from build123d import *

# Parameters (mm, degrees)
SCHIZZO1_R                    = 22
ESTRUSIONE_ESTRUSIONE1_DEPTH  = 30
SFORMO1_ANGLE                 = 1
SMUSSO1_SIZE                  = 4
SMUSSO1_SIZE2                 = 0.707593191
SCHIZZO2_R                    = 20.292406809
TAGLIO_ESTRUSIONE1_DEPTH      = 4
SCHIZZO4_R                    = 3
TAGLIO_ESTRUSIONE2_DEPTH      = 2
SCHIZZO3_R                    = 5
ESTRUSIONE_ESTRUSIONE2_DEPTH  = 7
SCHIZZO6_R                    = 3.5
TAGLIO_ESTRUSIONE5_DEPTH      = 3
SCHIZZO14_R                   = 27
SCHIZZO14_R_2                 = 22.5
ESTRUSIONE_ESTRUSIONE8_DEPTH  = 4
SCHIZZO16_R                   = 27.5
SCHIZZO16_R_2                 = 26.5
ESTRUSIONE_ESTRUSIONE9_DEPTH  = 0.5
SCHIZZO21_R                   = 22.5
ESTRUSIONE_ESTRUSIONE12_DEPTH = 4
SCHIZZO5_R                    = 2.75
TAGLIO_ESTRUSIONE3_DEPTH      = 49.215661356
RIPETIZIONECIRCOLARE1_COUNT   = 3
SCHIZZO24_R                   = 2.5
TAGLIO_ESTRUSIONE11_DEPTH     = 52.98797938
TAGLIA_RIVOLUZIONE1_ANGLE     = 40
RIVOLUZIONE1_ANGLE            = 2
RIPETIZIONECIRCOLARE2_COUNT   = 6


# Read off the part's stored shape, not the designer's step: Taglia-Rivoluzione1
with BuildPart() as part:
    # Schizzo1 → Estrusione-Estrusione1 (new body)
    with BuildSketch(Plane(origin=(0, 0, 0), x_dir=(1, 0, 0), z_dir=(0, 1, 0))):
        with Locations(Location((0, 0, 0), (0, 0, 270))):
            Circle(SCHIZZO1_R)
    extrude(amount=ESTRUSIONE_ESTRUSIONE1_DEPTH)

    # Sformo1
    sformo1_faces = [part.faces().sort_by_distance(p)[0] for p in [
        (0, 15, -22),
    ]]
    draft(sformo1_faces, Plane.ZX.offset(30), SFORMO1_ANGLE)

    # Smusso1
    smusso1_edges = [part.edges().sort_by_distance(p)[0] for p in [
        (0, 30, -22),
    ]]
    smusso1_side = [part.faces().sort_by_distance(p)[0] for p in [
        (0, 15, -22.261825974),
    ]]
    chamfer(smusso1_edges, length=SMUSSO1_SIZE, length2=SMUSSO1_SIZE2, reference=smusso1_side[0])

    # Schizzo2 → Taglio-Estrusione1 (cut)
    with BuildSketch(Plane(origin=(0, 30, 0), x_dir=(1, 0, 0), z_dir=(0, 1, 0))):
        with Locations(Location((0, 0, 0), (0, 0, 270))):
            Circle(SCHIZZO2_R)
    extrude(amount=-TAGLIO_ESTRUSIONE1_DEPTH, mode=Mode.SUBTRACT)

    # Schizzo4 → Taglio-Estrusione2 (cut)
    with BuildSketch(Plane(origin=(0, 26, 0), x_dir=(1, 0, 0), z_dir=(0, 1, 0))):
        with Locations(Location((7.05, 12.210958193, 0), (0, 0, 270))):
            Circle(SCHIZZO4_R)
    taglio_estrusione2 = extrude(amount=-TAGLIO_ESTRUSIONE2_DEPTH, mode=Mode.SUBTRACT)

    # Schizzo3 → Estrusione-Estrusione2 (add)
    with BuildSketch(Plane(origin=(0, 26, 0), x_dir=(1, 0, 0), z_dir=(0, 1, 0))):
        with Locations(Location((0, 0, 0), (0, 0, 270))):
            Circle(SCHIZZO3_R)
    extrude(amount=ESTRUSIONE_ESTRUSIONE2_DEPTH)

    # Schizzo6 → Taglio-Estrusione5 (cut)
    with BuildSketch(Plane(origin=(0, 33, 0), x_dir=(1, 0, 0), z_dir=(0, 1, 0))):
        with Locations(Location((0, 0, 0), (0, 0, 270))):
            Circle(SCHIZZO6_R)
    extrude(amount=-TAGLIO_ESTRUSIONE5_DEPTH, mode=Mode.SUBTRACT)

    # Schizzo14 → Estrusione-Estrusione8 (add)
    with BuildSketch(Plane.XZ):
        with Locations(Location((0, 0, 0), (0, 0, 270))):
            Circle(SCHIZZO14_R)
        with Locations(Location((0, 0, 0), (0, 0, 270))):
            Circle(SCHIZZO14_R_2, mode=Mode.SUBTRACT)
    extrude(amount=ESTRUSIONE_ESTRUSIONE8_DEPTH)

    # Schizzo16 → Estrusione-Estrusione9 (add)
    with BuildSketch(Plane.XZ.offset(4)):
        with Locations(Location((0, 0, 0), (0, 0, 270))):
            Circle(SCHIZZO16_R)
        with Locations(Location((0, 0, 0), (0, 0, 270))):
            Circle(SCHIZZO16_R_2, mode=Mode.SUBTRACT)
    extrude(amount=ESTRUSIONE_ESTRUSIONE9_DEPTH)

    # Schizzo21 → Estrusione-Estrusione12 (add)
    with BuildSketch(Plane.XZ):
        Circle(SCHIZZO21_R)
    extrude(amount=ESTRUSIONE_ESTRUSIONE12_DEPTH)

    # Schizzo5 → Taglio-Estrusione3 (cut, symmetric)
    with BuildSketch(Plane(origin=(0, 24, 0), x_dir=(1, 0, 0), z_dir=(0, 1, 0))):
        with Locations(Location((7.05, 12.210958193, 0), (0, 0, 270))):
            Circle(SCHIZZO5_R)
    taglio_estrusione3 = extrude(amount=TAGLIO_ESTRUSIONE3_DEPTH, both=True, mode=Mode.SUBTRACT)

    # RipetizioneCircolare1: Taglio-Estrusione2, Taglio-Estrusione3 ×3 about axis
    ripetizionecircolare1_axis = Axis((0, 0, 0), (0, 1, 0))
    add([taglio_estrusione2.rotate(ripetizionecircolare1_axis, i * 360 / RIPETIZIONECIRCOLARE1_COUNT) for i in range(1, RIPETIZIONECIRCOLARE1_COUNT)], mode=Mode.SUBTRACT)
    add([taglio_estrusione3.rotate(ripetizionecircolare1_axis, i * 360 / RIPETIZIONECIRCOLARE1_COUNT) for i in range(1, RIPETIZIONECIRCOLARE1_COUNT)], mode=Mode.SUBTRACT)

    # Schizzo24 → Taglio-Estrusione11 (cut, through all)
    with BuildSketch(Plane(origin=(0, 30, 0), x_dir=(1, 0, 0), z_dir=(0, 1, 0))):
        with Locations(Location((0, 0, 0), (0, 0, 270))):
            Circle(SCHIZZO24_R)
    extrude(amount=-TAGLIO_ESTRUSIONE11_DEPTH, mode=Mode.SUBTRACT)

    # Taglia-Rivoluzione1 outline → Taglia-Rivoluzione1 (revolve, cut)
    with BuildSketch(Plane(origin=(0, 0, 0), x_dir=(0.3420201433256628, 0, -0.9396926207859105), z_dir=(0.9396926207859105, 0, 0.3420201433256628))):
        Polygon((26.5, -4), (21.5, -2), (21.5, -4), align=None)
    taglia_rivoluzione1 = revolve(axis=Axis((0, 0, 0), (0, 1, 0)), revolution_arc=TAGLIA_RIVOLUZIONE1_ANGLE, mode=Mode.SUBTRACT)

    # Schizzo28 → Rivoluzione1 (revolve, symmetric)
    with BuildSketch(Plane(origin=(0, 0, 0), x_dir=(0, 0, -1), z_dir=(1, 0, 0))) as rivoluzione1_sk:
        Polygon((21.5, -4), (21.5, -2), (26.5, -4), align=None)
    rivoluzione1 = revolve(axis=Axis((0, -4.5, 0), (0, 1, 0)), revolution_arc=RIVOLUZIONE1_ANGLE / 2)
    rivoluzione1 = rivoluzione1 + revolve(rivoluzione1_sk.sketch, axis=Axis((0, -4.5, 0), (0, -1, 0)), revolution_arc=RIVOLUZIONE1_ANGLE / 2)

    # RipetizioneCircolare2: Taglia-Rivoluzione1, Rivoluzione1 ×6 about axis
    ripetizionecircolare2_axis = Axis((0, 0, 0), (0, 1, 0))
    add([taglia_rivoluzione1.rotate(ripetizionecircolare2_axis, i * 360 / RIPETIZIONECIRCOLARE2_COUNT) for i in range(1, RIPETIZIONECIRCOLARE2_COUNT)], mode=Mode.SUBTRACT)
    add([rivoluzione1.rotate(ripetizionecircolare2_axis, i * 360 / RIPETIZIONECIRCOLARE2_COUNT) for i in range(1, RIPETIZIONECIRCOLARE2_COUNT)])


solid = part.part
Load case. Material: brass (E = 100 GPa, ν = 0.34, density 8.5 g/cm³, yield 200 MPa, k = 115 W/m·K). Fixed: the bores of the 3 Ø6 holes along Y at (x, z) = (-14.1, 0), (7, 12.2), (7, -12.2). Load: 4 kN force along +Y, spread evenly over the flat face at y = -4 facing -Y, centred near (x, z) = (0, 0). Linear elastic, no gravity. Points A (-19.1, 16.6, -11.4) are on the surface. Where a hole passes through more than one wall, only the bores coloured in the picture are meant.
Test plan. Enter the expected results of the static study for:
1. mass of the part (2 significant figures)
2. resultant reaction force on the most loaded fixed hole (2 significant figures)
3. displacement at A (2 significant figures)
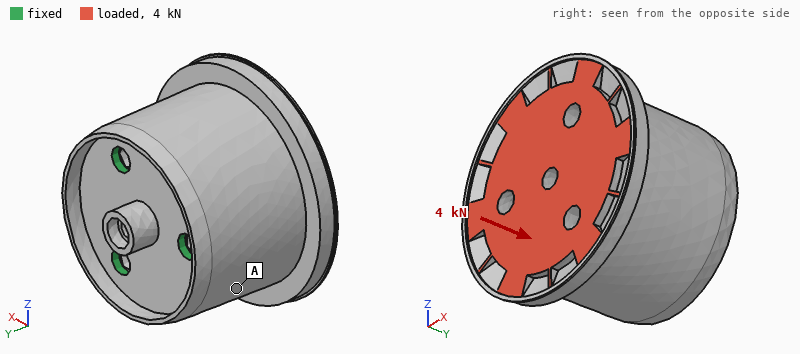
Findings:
410 g
1.3 kN
1.5 µm
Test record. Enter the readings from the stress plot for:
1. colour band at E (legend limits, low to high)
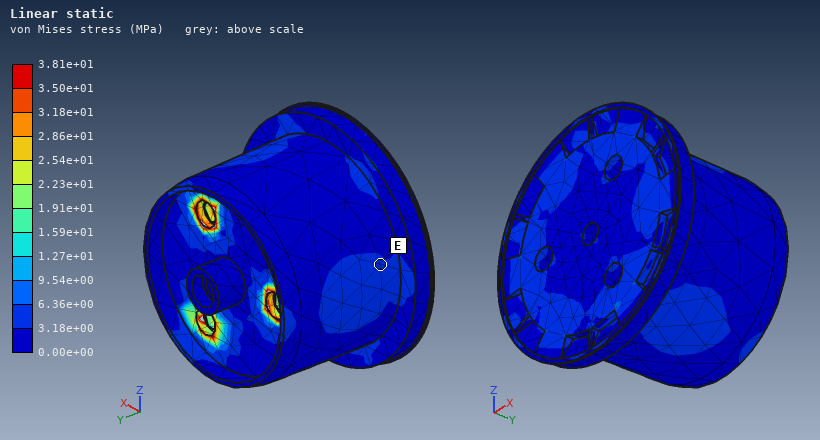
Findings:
3.18e+00 to 6.36e+00 MPa
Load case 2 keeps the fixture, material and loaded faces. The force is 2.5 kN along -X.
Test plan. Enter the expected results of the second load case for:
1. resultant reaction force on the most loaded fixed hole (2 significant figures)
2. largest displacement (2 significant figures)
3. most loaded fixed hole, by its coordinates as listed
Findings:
3.3 kN
14 µm
(-14.1, 0)
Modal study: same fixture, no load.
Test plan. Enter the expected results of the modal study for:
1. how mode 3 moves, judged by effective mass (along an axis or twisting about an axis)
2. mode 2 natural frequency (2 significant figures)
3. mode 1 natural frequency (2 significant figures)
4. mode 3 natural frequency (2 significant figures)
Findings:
twisting about Y
5900 Hz
5900 Hz
11 kHz
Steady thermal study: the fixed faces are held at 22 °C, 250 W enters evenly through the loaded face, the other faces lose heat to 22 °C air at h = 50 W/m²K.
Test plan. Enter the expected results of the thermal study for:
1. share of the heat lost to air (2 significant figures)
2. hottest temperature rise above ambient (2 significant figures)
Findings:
8.8 %
64 K
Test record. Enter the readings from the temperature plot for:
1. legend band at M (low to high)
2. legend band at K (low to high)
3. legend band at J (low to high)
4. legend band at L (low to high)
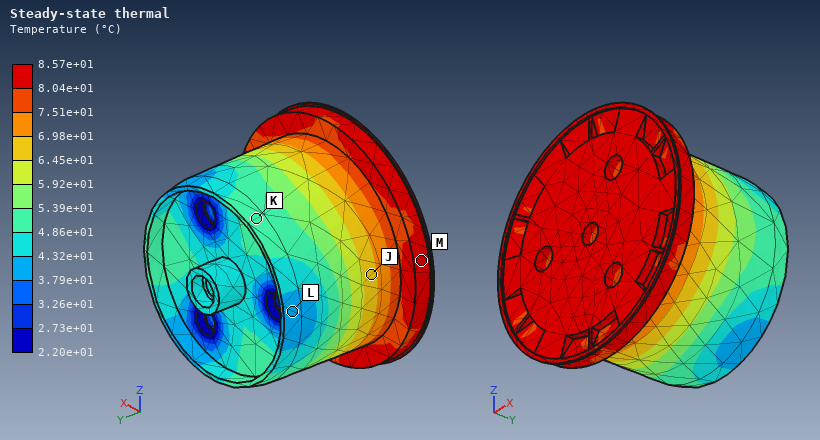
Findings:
8.04e+01 to 8.57e+01 °C
4.86e+01 to 5.39e+01 °C
6.45e+01 to 6.98e+01 °C
3.79e+01 to 4.32e+01 °C
